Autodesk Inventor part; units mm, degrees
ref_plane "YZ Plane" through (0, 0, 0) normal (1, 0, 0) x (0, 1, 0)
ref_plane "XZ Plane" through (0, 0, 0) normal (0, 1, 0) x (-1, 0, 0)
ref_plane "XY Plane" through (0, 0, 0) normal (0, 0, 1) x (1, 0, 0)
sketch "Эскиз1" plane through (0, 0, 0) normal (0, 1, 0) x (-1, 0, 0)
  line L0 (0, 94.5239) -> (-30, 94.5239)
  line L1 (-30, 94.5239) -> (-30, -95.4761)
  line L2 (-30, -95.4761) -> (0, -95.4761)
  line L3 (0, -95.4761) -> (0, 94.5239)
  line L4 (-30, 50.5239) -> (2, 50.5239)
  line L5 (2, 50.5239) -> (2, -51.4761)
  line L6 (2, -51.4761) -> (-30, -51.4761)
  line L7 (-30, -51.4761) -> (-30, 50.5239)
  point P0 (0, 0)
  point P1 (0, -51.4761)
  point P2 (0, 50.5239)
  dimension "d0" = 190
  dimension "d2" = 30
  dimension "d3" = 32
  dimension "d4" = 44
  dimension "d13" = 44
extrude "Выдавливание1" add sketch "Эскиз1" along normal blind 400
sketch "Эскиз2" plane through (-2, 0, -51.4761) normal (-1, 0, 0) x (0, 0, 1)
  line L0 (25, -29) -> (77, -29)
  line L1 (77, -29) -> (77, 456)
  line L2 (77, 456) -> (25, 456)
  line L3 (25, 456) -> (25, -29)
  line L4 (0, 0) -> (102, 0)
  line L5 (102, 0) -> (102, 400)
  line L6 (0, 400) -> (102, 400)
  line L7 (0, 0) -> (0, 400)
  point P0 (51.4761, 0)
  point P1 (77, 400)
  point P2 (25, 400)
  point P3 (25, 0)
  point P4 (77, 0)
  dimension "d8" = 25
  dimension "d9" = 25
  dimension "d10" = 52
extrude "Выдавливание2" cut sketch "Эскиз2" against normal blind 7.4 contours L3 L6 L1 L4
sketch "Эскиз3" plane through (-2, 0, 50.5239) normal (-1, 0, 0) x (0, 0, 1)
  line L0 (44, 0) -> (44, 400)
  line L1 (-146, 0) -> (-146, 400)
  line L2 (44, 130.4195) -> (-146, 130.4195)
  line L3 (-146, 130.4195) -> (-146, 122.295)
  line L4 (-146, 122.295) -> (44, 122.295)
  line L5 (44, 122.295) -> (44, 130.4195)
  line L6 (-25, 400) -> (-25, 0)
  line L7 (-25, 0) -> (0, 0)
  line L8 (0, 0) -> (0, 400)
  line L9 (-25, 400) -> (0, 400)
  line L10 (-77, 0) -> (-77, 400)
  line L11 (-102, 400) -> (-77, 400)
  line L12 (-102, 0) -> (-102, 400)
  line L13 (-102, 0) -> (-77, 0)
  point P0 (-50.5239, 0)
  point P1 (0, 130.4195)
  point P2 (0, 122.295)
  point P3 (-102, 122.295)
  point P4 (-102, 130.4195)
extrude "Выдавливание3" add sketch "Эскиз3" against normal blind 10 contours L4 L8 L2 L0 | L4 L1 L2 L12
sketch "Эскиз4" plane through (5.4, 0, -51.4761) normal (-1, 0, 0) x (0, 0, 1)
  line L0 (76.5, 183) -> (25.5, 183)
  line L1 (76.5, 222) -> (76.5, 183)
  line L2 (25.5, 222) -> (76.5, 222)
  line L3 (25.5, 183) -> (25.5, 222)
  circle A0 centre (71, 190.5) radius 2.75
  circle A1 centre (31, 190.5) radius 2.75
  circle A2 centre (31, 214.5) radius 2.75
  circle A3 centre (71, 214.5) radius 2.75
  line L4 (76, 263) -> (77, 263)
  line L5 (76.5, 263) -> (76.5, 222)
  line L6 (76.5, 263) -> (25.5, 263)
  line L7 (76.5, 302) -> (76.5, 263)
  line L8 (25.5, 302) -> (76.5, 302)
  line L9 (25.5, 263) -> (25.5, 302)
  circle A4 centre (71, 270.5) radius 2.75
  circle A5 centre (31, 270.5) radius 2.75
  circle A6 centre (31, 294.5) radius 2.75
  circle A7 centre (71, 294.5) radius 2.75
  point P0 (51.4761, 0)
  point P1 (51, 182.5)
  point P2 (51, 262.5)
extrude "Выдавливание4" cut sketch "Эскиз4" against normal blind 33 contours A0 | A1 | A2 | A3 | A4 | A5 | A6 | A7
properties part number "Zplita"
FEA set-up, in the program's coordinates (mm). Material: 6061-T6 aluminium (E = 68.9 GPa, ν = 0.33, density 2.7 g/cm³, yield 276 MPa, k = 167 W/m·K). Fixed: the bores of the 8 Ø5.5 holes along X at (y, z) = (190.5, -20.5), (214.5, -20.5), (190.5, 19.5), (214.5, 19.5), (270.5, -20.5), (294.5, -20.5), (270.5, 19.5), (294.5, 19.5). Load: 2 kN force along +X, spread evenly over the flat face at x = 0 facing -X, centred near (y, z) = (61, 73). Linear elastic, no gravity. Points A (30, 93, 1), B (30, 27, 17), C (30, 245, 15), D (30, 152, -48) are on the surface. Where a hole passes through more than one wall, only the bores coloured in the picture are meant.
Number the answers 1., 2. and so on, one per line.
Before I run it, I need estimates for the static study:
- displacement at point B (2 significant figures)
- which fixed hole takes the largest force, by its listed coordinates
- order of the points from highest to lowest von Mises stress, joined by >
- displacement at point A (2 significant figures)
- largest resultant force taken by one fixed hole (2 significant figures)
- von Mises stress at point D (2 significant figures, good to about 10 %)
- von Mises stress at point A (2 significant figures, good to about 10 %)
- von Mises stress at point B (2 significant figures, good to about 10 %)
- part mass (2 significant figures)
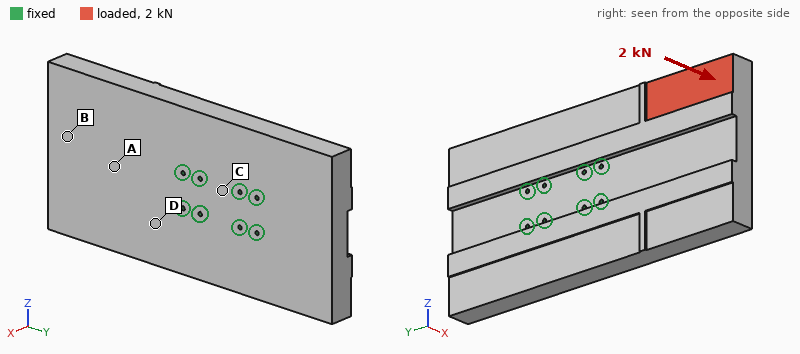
1. 0.11 mm
2. (190.5, 19.5)
3. D > A > B > C
4. 0.053 mm
5. 3.9 kN
6. 6.4 MPa
7. 4.3 MPa
8. 2.7 MPa
9. 6.0 kg
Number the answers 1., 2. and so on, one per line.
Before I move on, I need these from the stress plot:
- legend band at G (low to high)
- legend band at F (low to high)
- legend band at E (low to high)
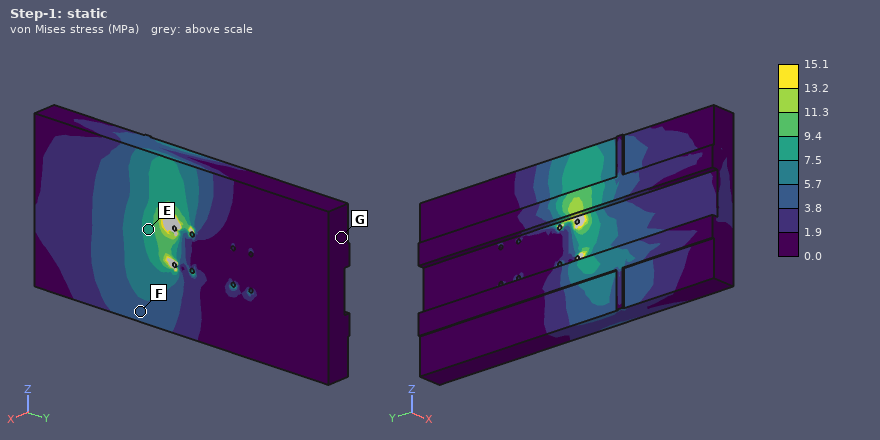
1. 0.0 to 1.9 MPa
2. 3.8 to 5.7 MPa
3. 7.5 to 9.4 MPa
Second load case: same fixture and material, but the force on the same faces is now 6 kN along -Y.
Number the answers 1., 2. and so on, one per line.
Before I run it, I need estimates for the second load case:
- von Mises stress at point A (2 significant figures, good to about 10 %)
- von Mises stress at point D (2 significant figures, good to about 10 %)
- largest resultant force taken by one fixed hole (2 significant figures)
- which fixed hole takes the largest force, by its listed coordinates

1. 2.1 MPa
2. 3.2 MPa
3. 3.3 kN
4. (190.5, 19.5)
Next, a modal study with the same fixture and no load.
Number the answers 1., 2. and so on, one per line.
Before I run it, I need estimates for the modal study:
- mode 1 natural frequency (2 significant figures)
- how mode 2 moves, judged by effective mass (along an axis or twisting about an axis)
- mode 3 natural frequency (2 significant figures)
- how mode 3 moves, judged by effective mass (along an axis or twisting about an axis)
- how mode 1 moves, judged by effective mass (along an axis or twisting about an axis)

1. 560 Hz
2. twisting about Y
3. 1500 Hz
4. along X
5. along X
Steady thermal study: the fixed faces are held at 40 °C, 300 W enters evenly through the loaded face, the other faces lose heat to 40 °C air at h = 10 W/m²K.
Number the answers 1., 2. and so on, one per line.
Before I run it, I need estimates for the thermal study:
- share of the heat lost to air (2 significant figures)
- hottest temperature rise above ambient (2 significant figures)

1. 10 %
2. 68 K
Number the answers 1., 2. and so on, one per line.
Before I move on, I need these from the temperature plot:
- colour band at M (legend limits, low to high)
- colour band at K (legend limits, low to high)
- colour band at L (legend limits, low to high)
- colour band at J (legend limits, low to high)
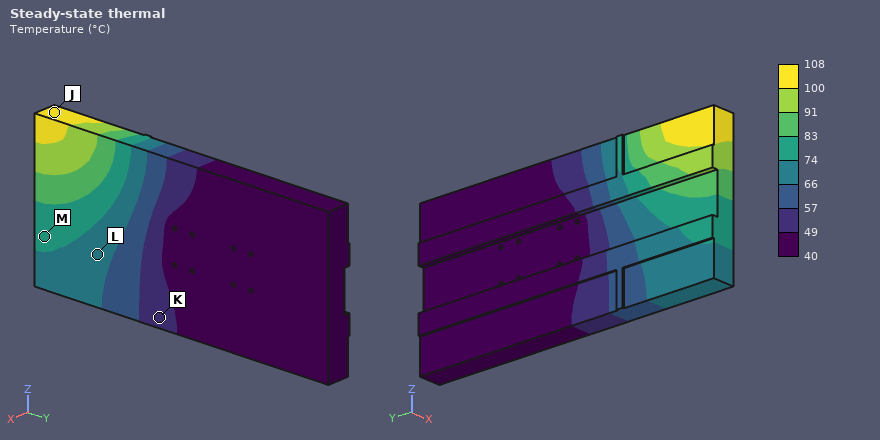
1. 74 to 83 °C
2. 49 to 57 °C
3. 66 to 74 °C
4. 100 to 108 °C
